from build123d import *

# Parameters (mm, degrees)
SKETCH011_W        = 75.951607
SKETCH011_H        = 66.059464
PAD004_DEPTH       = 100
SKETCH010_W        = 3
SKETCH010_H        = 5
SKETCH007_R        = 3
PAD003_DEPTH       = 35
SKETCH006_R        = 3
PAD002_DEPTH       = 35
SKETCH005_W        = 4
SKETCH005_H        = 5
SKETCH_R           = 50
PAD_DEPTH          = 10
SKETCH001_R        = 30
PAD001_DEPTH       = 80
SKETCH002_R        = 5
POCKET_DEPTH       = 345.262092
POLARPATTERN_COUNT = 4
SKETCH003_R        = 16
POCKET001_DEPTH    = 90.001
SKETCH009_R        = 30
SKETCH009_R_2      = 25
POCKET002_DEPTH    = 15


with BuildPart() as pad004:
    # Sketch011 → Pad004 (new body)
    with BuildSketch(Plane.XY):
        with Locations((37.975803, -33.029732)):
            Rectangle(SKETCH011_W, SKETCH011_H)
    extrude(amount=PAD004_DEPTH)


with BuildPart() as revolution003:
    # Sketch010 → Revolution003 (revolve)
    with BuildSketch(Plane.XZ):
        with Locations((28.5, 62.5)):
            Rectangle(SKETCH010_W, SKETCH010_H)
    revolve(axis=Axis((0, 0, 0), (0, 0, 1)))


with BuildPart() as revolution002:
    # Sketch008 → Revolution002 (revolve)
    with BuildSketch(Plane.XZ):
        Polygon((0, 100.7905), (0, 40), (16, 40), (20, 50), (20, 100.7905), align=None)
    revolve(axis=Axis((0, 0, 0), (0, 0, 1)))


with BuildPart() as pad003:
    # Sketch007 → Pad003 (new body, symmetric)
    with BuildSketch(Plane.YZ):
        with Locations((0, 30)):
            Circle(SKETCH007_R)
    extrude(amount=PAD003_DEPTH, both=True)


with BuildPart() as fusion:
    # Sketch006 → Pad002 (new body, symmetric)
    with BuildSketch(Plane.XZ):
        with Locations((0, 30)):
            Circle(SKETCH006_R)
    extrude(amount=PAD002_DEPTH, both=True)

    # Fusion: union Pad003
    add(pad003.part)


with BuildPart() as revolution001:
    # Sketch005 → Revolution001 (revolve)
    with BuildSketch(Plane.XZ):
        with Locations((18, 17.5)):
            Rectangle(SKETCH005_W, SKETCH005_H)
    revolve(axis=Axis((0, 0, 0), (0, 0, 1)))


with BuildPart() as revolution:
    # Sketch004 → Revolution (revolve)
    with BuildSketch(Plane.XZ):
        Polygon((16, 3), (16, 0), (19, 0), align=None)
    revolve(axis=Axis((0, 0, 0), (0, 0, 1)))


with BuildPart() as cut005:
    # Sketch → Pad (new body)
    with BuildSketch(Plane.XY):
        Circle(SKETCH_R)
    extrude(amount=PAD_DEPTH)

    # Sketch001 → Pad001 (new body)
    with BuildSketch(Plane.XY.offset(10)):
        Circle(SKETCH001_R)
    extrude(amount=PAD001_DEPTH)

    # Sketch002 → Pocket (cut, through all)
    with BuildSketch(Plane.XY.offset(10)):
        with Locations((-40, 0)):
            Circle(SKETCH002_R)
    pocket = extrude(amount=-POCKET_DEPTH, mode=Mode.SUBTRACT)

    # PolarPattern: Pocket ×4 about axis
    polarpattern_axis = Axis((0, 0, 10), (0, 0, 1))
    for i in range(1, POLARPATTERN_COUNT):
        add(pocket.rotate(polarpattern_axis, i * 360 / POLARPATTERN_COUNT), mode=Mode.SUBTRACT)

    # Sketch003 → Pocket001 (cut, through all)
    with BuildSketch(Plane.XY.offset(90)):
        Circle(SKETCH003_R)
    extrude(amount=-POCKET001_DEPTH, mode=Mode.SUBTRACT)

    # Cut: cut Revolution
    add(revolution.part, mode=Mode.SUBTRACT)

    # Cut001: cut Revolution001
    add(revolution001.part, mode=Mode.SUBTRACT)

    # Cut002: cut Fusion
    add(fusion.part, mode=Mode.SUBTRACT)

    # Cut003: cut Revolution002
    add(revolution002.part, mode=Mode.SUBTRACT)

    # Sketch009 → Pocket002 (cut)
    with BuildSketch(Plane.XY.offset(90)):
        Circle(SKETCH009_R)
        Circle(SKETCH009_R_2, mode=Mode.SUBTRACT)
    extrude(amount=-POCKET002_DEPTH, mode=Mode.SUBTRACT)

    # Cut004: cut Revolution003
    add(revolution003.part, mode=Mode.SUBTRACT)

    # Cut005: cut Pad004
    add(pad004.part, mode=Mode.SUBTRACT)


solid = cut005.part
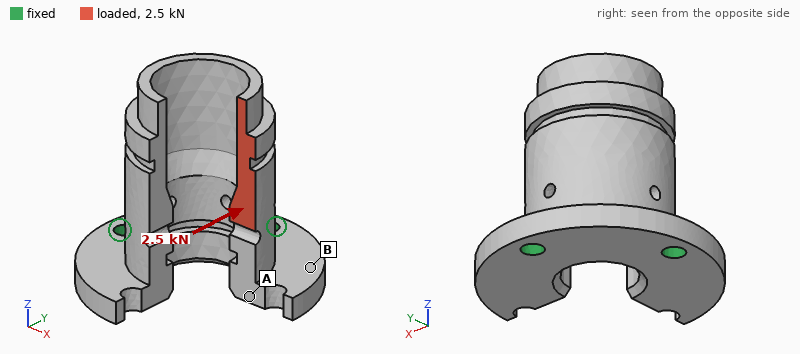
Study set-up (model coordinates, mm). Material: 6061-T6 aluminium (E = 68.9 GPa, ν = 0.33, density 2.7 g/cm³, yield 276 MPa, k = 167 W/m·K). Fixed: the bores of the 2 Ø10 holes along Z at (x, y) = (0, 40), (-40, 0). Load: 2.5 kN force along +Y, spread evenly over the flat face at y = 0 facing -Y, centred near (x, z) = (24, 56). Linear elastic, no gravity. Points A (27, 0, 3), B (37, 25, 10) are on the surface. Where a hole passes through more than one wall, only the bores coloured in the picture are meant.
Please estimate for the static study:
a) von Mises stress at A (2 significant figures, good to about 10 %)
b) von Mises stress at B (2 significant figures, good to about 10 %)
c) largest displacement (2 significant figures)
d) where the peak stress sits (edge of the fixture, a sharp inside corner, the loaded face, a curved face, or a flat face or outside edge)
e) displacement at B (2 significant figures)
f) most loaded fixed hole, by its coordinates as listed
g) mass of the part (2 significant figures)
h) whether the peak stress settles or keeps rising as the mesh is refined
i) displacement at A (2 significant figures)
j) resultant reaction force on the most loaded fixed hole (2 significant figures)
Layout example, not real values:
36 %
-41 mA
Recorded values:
7.8 MPa
15 MPa
0.40 mm
edge of the fixture
0.067 mm
(0, 40)
380 g
keeps rising
0.14 mm
3.1 kN
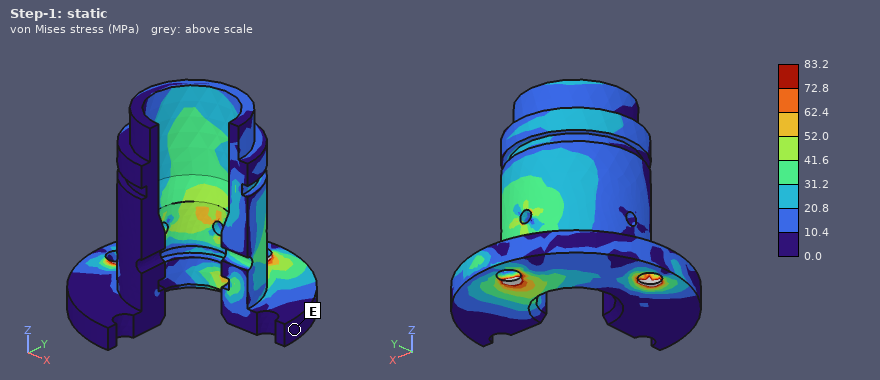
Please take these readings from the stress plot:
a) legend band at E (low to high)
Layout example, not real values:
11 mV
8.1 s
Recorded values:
0.0 to 10.4 MPa
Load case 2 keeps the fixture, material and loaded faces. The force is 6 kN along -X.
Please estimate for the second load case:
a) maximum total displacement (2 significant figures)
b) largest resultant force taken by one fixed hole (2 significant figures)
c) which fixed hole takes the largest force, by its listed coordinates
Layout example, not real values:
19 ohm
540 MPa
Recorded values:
0.68 mm
6.2 kN
(-40, 0)
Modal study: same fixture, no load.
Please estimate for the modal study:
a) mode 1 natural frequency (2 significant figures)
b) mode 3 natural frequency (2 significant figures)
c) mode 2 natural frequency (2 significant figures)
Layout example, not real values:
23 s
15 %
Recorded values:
1300 Hz
3200 Hz
2400 Hz
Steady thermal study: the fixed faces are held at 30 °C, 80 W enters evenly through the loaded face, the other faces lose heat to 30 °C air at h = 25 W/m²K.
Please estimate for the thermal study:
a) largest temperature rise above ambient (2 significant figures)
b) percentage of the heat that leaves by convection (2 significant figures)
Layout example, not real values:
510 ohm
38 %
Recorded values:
52 K
16 %
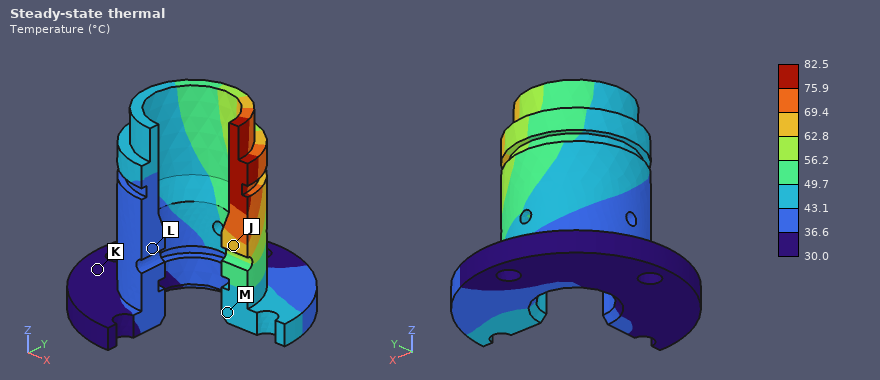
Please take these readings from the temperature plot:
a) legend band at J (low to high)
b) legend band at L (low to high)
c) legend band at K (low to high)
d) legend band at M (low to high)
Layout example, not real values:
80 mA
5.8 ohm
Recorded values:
62.8 to 69.4 °C
36.6 to 43.1 °C
30.0 to 36.6 °C
43.1 to 49.7 °C
